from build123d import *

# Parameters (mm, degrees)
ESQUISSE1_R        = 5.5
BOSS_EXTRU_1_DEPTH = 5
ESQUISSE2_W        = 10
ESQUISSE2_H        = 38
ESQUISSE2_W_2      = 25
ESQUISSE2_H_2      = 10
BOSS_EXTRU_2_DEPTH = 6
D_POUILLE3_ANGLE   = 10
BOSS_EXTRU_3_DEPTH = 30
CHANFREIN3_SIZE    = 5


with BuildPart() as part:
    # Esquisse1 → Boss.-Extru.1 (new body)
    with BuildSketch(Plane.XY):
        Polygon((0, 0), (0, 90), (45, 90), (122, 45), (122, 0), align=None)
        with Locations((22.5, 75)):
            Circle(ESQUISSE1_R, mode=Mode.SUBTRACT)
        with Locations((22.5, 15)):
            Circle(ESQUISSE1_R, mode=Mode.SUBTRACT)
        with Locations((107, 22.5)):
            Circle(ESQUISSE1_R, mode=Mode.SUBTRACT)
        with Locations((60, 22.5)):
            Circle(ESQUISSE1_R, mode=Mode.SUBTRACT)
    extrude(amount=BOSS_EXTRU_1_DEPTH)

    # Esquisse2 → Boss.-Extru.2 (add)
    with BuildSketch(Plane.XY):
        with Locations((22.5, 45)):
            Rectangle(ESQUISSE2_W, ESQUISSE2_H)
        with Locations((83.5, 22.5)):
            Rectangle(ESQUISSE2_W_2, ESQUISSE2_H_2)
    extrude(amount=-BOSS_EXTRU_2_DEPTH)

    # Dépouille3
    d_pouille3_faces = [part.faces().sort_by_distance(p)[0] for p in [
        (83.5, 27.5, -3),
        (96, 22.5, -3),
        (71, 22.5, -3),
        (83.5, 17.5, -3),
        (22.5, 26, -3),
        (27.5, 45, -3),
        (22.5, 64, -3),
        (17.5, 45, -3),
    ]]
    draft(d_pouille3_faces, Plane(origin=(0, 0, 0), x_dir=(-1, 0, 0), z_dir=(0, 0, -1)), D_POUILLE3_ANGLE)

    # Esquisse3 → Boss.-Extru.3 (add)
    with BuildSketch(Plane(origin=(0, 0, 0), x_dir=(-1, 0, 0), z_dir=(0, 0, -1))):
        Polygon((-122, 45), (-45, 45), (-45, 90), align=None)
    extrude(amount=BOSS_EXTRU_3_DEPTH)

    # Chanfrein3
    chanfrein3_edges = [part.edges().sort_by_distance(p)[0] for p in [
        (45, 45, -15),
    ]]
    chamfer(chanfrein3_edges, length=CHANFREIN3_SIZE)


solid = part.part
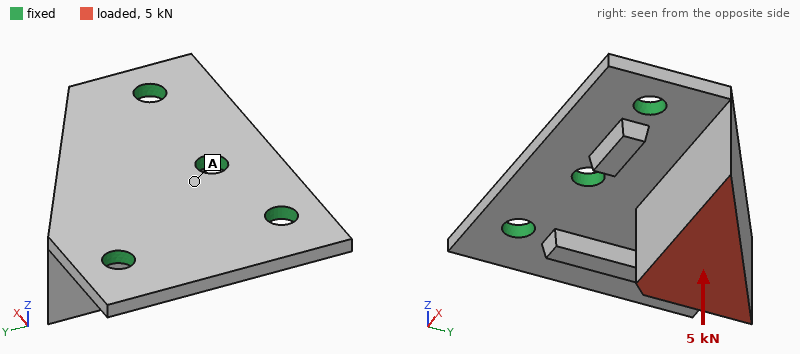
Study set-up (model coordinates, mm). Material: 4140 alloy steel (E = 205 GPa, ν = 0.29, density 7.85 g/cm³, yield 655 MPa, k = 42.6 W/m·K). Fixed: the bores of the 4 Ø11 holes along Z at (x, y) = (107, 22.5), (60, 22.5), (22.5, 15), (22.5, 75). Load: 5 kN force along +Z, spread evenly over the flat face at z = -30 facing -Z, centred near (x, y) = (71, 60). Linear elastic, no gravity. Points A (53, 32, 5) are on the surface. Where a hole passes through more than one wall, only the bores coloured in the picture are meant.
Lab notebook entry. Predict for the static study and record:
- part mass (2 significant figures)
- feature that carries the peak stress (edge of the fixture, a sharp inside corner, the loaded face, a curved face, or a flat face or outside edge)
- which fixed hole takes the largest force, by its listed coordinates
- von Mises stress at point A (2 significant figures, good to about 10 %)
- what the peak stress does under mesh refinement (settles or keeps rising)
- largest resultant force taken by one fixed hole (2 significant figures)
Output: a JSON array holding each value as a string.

["780 g", "edge of the fixture", "(22.5, 75)", "32 MPa", "keeps rising", "2.8 kN"]
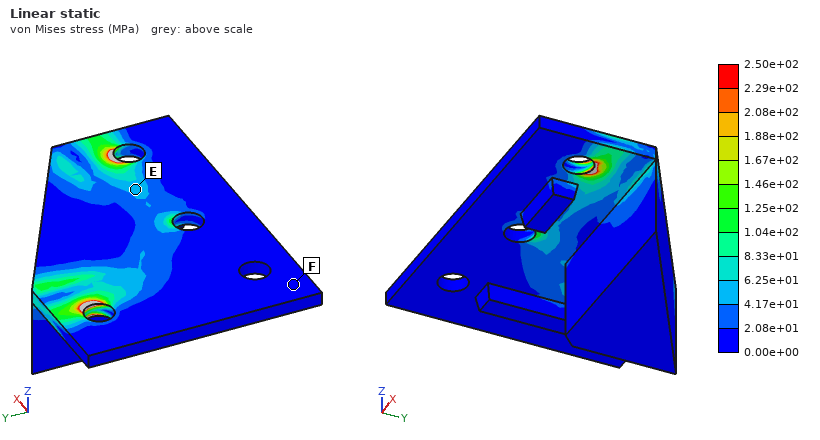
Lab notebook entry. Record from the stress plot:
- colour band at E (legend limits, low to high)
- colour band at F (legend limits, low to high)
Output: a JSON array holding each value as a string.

["4.17e+01 to 6.25e+01 MPa", "0.00e+00 to 2.08e+01 MPa"]
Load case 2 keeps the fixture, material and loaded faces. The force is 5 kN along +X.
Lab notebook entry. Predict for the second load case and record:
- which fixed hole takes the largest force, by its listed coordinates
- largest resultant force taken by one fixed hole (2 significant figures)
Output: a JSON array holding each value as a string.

["(107, 22.5)", "3.3 kN"]
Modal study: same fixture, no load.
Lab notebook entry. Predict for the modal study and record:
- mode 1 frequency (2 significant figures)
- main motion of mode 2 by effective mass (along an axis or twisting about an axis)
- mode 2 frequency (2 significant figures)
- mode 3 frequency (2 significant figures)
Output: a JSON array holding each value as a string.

["1800 Hz", "along X", "4000 Hz", "4200 Hz"]
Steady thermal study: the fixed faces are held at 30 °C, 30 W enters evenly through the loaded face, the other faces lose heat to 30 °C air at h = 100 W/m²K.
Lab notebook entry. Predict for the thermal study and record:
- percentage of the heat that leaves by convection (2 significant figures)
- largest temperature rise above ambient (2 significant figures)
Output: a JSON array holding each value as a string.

["62 %", "25 K"]
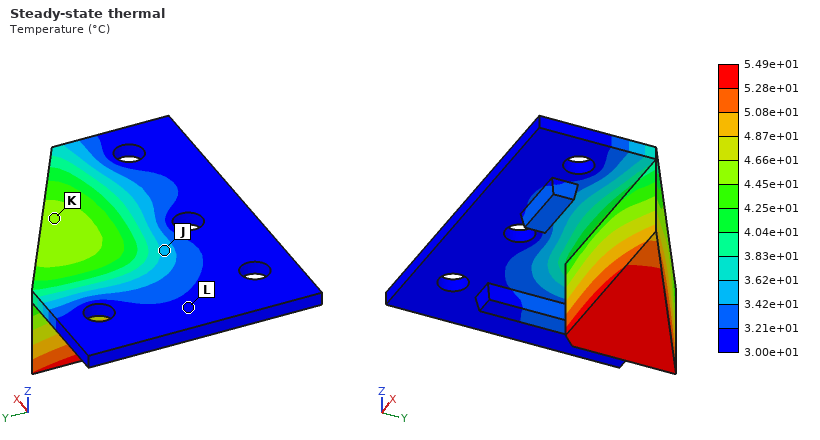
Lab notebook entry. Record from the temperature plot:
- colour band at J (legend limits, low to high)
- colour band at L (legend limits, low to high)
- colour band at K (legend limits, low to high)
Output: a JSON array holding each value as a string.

["3.42e+01 to 3.62e+01 °C", "3.00e+01 to 3.21e+01 °C", "4.45e+01 to 4.66e+01 °C"]
